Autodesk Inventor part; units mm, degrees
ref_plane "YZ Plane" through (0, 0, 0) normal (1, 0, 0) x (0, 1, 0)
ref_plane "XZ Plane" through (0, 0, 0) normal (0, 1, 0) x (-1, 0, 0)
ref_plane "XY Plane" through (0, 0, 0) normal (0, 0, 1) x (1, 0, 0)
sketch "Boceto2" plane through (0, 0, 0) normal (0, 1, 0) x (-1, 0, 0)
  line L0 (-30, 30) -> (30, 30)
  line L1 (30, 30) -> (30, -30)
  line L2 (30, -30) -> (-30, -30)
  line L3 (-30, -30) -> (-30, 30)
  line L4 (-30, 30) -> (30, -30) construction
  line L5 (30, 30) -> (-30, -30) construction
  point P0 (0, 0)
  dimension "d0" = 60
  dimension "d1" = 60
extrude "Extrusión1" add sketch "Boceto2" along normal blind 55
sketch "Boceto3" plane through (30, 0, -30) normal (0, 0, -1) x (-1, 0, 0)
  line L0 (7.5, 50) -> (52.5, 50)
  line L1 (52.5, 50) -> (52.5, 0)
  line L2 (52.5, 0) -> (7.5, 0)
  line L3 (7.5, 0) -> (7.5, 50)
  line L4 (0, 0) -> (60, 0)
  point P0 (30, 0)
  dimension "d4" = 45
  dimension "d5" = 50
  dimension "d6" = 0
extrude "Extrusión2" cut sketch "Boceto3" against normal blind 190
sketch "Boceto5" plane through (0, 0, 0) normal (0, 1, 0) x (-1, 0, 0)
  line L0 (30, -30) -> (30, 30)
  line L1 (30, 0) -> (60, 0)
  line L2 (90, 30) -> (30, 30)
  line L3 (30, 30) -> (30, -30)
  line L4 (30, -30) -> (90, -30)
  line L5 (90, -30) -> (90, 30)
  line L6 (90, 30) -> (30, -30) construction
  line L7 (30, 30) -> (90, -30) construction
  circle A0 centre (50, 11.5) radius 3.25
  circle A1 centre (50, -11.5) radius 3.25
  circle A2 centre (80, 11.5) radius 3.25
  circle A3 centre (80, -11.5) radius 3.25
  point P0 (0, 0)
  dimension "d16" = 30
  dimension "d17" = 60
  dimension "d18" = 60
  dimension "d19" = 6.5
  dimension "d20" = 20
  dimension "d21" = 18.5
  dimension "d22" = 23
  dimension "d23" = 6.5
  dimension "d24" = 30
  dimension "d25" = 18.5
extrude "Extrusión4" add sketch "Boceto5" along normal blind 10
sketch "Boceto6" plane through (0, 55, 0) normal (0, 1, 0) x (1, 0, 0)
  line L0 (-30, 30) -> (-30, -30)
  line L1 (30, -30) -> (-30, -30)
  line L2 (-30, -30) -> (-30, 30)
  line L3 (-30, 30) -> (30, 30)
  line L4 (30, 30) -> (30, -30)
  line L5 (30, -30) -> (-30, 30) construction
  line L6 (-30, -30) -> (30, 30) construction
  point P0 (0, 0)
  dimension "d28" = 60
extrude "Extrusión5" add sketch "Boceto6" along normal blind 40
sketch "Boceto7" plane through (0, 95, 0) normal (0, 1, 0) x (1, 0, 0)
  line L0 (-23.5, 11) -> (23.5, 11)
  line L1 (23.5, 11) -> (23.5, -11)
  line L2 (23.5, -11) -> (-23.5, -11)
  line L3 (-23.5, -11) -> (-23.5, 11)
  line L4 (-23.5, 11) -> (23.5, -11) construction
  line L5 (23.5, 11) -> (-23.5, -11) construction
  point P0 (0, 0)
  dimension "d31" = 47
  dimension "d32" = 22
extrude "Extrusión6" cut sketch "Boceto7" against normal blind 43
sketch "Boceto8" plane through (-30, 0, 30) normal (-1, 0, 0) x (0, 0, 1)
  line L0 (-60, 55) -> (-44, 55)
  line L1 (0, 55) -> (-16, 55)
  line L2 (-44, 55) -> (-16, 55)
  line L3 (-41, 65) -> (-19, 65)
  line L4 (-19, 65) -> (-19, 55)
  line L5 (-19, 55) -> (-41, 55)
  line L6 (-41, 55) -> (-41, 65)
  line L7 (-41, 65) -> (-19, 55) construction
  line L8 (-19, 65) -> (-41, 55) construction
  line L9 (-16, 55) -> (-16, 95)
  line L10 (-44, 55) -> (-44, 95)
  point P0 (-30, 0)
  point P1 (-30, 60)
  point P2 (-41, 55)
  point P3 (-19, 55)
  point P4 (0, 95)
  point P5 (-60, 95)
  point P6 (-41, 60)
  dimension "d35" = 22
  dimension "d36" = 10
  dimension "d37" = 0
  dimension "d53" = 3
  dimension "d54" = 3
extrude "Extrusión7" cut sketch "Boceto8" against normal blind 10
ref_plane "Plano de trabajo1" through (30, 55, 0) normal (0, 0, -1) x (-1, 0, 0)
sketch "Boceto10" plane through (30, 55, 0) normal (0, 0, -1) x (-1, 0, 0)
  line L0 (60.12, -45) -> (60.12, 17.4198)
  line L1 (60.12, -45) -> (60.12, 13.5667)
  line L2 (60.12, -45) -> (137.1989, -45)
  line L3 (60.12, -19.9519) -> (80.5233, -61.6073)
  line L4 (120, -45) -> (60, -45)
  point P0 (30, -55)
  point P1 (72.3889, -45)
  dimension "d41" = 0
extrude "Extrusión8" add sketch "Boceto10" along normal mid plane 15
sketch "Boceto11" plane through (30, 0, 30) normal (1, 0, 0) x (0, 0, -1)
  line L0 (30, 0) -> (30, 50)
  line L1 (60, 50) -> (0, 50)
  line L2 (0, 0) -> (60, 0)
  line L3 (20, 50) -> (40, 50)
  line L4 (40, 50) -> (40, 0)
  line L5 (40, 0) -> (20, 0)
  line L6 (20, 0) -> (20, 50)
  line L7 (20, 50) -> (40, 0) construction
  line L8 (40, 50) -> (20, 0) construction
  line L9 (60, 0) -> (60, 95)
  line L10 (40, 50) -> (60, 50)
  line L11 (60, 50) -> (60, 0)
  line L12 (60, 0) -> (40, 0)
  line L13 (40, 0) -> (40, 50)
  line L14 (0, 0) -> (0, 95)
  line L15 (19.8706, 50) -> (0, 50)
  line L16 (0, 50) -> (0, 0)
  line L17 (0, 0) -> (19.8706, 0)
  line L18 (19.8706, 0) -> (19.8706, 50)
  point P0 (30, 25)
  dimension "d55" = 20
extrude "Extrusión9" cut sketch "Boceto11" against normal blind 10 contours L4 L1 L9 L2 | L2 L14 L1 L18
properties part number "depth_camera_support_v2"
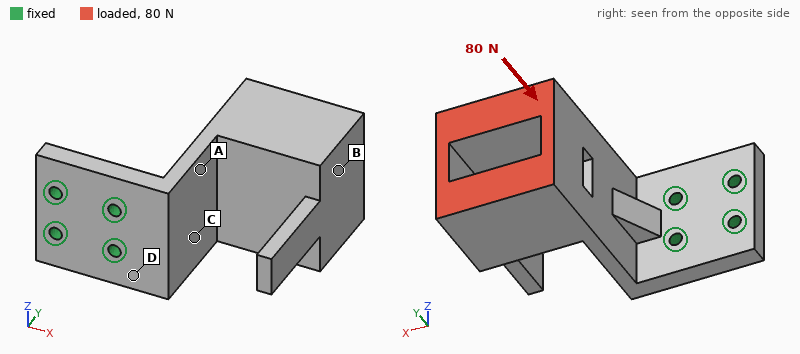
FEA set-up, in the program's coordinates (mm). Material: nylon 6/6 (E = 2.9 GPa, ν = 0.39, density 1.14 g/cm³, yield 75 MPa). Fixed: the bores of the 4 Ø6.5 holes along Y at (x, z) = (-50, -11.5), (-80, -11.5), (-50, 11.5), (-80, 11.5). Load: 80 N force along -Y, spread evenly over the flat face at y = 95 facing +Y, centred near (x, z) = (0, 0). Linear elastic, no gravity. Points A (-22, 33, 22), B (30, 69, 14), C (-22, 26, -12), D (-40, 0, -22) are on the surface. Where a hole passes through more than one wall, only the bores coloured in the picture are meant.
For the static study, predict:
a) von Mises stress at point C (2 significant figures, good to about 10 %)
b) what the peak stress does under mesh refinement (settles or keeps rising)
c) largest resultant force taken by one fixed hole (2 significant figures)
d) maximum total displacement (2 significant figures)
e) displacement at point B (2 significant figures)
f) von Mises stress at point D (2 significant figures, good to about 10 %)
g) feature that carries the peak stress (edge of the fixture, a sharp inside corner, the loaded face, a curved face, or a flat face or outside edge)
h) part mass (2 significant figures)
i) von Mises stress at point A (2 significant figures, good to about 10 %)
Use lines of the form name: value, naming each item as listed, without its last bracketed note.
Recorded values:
von Mises stress at point C: 3.5 MPa
what the peak stress does under mesh refinement: keeps rising
largest resultant force taken by one fixed hole: 59 N
maximum total displacement: 1.8 mm
displacement at point B: 1.5 mm
von Mises stress at point D: 2.5 MPa
feature that carries the peak stress: edge of the fixture
part mass: 210 g
von Mises stress at point A: 3.9 MPa
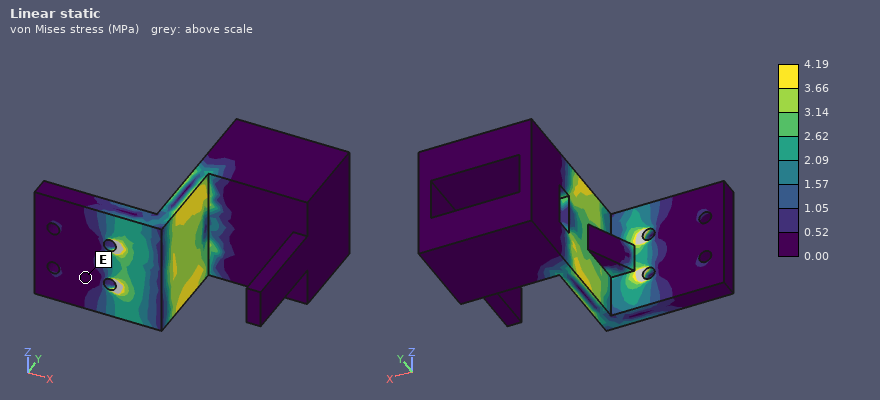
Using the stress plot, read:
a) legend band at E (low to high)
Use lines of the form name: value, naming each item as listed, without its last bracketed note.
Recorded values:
legend band at E: 0.00 to 0.52 MPa
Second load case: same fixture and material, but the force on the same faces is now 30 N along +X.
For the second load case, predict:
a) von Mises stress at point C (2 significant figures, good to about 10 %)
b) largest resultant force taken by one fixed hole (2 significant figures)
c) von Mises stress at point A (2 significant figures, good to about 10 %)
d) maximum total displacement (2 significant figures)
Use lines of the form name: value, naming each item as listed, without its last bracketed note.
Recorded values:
von Mises stress at point C: 3.2 MPa
largest resultant force taken by one fixed hole: 24 N
von Mises stress at point A: 3.2 MPa
maximum total displacement: 1.7 mm
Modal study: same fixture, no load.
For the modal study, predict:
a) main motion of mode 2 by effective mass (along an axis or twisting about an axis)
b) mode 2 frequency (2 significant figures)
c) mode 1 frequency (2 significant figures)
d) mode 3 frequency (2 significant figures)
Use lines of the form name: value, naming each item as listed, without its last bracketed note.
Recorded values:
main motion of mode 2 by effective mass: along Z
mode 2 frequency: 190 Hz
mode 1 frequency: 76 Hz
mode 3 frequency: 310 Hz
